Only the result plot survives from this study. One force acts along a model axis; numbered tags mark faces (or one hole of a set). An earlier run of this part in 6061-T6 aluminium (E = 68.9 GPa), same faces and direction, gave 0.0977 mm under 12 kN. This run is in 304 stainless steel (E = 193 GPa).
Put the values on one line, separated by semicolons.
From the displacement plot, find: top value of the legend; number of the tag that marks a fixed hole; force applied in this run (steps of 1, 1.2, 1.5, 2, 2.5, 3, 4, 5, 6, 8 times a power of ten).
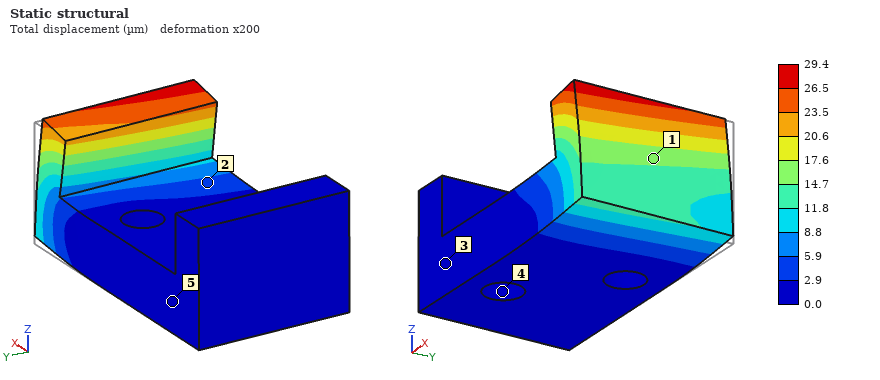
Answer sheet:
29.4 µm; 4; 10 kN
